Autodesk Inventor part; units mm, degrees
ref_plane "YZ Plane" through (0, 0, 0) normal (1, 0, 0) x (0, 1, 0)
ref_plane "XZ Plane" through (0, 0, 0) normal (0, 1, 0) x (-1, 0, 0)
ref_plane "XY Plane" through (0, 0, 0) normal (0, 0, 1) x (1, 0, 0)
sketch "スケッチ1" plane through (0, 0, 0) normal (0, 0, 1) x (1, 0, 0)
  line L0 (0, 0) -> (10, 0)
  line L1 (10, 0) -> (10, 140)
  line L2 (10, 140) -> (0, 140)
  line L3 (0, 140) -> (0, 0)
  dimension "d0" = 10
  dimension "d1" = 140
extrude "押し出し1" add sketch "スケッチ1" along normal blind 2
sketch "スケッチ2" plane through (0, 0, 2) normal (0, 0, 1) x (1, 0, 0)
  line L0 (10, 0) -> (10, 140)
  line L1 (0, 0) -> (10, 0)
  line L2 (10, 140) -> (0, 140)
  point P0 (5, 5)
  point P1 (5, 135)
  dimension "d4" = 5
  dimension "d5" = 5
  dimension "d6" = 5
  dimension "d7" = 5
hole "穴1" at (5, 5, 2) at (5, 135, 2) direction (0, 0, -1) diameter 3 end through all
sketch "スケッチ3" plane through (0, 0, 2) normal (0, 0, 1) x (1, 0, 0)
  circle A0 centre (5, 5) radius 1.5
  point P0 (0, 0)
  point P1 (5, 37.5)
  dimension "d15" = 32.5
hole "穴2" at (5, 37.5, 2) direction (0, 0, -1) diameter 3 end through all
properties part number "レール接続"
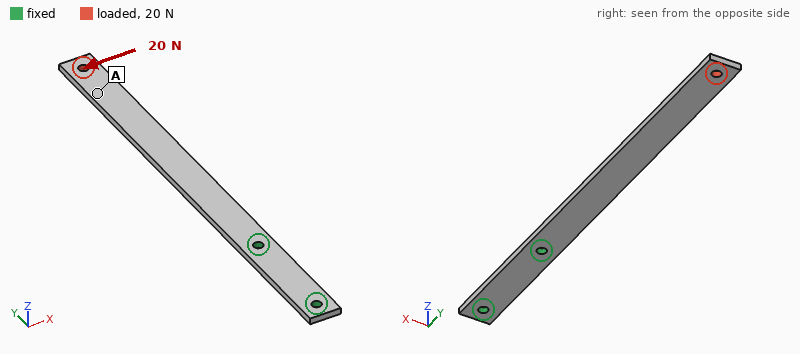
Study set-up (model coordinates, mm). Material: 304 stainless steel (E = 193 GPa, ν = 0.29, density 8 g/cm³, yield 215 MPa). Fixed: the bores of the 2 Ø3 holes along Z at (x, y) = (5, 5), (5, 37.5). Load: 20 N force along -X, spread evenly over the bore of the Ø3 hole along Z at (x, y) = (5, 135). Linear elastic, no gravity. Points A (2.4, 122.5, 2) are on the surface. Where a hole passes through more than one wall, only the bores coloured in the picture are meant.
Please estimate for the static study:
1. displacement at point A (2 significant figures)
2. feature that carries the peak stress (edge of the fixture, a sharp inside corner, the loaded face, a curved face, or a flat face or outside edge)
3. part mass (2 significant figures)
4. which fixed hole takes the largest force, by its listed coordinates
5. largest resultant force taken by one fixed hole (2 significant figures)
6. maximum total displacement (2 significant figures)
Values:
0.18 mm
edge of the fixture
22 g
(5, 37.5)
48 N
0.23 mm
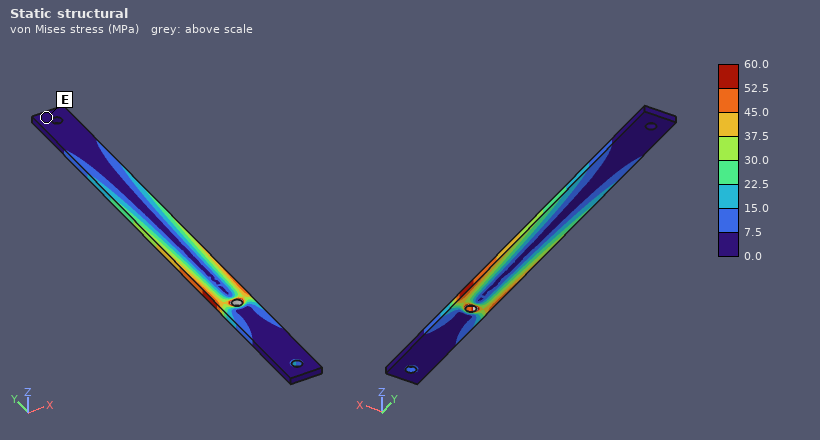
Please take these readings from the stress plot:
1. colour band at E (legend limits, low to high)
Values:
0.0 to 7.5 MPa
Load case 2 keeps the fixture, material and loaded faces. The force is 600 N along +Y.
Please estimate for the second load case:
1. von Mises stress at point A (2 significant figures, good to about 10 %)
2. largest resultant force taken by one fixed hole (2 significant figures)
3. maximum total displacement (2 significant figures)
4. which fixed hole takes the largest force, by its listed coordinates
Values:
30 MPa
580 N
16 µm
(5, 37.5)
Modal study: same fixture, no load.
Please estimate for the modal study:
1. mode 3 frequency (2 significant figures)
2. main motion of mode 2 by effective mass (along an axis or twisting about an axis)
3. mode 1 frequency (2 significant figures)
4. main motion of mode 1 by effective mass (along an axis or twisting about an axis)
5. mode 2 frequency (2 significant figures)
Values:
970 Hz
along X
160 Hz
along Z
710 Hz
